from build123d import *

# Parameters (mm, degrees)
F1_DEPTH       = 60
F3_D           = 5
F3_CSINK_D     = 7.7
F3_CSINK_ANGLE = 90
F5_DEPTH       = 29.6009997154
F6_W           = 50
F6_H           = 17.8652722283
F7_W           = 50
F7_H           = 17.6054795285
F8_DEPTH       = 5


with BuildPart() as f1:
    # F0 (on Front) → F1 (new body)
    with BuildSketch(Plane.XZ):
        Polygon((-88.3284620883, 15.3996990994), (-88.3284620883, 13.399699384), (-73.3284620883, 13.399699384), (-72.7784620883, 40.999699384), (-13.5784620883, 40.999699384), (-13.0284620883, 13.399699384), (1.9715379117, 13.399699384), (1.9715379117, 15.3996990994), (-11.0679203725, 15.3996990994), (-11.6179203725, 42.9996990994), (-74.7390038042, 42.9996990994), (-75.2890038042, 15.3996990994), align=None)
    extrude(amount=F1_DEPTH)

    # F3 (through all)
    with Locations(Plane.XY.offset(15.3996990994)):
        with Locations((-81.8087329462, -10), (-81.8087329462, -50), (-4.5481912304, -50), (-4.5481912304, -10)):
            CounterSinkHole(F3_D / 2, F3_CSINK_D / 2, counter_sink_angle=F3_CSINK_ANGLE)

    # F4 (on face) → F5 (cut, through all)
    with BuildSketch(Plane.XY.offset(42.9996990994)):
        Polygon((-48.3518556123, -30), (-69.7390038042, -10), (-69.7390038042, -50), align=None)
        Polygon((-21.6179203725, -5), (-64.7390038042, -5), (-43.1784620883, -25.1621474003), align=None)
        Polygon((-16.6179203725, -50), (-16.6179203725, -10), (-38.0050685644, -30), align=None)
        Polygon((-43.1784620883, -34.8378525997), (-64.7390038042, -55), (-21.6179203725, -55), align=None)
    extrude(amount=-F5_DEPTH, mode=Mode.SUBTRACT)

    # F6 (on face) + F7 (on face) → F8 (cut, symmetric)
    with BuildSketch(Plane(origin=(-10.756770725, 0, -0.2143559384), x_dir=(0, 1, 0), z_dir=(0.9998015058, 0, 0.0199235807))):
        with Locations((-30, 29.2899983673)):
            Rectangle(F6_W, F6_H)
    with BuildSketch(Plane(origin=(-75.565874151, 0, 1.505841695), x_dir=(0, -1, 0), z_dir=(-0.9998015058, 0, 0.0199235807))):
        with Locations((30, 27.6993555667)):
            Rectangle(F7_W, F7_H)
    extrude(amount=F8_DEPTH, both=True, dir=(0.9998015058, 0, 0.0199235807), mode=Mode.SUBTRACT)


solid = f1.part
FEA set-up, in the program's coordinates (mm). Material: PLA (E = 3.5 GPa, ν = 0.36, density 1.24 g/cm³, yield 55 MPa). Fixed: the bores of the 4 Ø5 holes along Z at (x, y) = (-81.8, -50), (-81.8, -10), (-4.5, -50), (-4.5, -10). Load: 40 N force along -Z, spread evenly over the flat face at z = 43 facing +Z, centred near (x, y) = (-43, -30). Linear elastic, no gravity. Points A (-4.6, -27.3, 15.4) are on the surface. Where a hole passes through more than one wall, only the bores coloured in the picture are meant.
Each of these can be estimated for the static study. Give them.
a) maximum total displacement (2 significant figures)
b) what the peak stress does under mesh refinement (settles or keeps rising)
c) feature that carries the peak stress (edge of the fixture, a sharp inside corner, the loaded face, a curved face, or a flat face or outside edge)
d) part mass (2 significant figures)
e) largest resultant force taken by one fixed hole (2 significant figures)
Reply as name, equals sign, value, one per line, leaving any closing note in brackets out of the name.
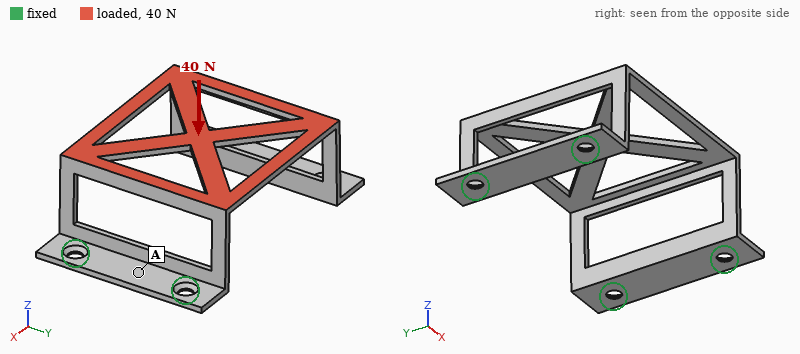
maximum total displacement = 1.2 mm
what the peak stress does under mesh refinement = keeps rising
feature that carries the peak stress = a sharp inside corner
part mass = 13 g
largest resultant force taken by one fixed hole = 14 N
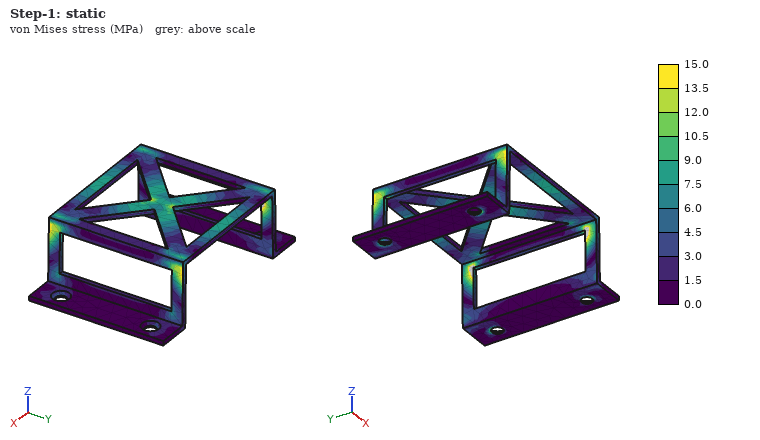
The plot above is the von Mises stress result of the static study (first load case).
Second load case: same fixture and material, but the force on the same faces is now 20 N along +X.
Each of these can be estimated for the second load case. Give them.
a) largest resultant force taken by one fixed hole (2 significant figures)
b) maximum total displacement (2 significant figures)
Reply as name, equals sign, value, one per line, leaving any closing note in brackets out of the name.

largest resultant force taken by one fixed hole = 6.3 N
maximum total displacement = 1.1 mm
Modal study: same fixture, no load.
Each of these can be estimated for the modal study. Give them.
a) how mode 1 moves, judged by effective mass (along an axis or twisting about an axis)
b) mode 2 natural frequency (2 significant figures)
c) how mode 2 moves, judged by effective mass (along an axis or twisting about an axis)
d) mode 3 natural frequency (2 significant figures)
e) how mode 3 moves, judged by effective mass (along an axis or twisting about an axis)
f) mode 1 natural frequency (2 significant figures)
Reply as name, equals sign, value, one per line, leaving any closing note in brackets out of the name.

how mode 1 moves, judged by effective mass = along X
mode 2 natural frequency = 500 Hz
how mode 2 moves, judged by effective mass = along Z
mode 3 natural frequency = 640 Hz
how mode 3 moves, judged by effective mass = along Y
mode 1 natural frequency = 280 Hz
